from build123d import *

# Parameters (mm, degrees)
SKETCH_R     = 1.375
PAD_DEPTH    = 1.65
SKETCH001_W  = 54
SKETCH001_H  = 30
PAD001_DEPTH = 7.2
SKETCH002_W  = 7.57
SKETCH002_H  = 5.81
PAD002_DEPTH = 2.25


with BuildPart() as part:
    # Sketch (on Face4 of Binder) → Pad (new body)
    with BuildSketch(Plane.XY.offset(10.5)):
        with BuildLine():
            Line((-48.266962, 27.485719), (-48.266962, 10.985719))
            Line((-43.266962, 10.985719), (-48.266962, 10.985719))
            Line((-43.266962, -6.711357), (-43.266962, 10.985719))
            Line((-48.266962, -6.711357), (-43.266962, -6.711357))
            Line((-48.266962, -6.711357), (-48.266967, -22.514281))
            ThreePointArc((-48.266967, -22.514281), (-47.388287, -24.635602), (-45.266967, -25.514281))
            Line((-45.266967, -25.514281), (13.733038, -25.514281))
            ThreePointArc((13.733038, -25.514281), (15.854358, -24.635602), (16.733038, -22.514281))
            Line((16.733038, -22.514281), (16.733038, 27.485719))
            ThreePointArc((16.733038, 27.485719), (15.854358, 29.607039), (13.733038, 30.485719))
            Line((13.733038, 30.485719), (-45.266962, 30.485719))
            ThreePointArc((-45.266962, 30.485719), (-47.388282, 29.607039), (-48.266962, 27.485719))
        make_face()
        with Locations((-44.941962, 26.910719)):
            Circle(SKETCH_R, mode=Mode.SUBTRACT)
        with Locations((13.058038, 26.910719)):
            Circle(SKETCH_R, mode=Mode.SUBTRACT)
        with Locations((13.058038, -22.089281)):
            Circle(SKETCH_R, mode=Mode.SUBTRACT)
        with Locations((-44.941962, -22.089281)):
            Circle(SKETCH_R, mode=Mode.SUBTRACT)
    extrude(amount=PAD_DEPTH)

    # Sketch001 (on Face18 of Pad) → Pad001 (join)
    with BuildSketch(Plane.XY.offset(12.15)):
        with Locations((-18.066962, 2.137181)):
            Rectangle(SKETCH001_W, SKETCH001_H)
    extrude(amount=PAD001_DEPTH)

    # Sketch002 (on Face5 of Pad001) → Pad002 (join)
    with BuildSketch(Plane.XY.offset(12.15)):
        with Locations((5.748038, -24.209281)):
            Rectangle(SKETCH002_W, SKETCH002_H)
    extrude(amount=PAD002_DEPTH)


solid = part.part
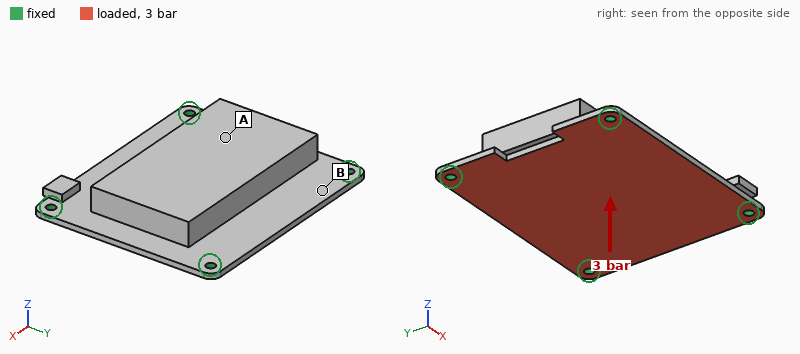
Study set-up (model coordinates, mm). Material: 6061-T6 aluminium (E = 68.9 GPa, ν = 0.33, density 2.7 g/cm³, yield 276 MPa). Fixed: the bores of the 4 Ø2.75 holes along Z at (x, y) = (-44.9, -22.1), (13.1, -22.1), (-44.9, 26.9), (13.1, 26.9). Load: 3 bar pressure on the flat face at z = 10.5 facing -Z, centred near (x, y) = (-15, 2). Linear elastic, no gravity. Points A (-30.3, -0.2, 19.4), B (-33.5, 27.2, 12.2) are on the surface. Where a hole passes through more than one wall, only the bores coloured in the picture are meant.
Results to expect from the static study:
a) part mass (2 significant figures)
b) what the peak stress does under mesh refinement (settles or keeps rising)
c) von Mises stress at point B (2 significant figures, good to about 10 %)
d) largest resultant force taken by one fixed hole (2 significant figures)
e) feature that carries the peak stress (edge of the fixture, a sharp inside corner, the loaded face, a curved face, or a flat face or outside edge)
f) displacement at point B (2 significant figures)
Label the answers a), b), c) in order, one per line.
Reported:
a) 47 g
b) keeps rising
c) 35 MPa
d) 310 N
e) edge of the fixture
f) 0.061 mm
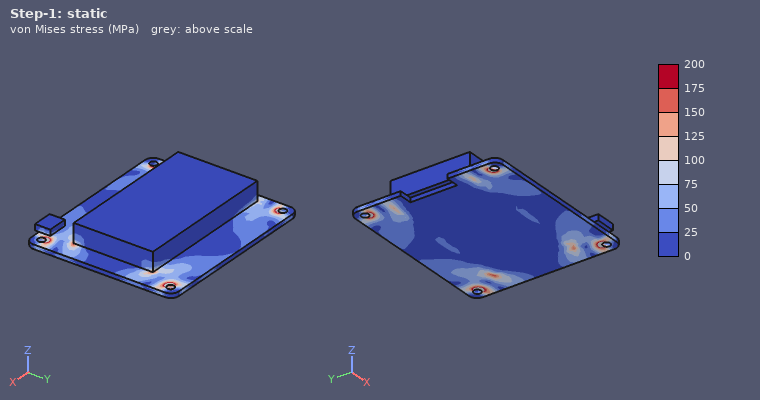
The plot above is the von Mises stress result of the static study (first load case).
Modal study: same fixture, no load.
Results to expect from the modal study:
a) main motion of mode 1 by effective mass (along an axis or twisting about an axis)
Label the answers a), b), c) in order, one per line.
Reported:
a) along Z
